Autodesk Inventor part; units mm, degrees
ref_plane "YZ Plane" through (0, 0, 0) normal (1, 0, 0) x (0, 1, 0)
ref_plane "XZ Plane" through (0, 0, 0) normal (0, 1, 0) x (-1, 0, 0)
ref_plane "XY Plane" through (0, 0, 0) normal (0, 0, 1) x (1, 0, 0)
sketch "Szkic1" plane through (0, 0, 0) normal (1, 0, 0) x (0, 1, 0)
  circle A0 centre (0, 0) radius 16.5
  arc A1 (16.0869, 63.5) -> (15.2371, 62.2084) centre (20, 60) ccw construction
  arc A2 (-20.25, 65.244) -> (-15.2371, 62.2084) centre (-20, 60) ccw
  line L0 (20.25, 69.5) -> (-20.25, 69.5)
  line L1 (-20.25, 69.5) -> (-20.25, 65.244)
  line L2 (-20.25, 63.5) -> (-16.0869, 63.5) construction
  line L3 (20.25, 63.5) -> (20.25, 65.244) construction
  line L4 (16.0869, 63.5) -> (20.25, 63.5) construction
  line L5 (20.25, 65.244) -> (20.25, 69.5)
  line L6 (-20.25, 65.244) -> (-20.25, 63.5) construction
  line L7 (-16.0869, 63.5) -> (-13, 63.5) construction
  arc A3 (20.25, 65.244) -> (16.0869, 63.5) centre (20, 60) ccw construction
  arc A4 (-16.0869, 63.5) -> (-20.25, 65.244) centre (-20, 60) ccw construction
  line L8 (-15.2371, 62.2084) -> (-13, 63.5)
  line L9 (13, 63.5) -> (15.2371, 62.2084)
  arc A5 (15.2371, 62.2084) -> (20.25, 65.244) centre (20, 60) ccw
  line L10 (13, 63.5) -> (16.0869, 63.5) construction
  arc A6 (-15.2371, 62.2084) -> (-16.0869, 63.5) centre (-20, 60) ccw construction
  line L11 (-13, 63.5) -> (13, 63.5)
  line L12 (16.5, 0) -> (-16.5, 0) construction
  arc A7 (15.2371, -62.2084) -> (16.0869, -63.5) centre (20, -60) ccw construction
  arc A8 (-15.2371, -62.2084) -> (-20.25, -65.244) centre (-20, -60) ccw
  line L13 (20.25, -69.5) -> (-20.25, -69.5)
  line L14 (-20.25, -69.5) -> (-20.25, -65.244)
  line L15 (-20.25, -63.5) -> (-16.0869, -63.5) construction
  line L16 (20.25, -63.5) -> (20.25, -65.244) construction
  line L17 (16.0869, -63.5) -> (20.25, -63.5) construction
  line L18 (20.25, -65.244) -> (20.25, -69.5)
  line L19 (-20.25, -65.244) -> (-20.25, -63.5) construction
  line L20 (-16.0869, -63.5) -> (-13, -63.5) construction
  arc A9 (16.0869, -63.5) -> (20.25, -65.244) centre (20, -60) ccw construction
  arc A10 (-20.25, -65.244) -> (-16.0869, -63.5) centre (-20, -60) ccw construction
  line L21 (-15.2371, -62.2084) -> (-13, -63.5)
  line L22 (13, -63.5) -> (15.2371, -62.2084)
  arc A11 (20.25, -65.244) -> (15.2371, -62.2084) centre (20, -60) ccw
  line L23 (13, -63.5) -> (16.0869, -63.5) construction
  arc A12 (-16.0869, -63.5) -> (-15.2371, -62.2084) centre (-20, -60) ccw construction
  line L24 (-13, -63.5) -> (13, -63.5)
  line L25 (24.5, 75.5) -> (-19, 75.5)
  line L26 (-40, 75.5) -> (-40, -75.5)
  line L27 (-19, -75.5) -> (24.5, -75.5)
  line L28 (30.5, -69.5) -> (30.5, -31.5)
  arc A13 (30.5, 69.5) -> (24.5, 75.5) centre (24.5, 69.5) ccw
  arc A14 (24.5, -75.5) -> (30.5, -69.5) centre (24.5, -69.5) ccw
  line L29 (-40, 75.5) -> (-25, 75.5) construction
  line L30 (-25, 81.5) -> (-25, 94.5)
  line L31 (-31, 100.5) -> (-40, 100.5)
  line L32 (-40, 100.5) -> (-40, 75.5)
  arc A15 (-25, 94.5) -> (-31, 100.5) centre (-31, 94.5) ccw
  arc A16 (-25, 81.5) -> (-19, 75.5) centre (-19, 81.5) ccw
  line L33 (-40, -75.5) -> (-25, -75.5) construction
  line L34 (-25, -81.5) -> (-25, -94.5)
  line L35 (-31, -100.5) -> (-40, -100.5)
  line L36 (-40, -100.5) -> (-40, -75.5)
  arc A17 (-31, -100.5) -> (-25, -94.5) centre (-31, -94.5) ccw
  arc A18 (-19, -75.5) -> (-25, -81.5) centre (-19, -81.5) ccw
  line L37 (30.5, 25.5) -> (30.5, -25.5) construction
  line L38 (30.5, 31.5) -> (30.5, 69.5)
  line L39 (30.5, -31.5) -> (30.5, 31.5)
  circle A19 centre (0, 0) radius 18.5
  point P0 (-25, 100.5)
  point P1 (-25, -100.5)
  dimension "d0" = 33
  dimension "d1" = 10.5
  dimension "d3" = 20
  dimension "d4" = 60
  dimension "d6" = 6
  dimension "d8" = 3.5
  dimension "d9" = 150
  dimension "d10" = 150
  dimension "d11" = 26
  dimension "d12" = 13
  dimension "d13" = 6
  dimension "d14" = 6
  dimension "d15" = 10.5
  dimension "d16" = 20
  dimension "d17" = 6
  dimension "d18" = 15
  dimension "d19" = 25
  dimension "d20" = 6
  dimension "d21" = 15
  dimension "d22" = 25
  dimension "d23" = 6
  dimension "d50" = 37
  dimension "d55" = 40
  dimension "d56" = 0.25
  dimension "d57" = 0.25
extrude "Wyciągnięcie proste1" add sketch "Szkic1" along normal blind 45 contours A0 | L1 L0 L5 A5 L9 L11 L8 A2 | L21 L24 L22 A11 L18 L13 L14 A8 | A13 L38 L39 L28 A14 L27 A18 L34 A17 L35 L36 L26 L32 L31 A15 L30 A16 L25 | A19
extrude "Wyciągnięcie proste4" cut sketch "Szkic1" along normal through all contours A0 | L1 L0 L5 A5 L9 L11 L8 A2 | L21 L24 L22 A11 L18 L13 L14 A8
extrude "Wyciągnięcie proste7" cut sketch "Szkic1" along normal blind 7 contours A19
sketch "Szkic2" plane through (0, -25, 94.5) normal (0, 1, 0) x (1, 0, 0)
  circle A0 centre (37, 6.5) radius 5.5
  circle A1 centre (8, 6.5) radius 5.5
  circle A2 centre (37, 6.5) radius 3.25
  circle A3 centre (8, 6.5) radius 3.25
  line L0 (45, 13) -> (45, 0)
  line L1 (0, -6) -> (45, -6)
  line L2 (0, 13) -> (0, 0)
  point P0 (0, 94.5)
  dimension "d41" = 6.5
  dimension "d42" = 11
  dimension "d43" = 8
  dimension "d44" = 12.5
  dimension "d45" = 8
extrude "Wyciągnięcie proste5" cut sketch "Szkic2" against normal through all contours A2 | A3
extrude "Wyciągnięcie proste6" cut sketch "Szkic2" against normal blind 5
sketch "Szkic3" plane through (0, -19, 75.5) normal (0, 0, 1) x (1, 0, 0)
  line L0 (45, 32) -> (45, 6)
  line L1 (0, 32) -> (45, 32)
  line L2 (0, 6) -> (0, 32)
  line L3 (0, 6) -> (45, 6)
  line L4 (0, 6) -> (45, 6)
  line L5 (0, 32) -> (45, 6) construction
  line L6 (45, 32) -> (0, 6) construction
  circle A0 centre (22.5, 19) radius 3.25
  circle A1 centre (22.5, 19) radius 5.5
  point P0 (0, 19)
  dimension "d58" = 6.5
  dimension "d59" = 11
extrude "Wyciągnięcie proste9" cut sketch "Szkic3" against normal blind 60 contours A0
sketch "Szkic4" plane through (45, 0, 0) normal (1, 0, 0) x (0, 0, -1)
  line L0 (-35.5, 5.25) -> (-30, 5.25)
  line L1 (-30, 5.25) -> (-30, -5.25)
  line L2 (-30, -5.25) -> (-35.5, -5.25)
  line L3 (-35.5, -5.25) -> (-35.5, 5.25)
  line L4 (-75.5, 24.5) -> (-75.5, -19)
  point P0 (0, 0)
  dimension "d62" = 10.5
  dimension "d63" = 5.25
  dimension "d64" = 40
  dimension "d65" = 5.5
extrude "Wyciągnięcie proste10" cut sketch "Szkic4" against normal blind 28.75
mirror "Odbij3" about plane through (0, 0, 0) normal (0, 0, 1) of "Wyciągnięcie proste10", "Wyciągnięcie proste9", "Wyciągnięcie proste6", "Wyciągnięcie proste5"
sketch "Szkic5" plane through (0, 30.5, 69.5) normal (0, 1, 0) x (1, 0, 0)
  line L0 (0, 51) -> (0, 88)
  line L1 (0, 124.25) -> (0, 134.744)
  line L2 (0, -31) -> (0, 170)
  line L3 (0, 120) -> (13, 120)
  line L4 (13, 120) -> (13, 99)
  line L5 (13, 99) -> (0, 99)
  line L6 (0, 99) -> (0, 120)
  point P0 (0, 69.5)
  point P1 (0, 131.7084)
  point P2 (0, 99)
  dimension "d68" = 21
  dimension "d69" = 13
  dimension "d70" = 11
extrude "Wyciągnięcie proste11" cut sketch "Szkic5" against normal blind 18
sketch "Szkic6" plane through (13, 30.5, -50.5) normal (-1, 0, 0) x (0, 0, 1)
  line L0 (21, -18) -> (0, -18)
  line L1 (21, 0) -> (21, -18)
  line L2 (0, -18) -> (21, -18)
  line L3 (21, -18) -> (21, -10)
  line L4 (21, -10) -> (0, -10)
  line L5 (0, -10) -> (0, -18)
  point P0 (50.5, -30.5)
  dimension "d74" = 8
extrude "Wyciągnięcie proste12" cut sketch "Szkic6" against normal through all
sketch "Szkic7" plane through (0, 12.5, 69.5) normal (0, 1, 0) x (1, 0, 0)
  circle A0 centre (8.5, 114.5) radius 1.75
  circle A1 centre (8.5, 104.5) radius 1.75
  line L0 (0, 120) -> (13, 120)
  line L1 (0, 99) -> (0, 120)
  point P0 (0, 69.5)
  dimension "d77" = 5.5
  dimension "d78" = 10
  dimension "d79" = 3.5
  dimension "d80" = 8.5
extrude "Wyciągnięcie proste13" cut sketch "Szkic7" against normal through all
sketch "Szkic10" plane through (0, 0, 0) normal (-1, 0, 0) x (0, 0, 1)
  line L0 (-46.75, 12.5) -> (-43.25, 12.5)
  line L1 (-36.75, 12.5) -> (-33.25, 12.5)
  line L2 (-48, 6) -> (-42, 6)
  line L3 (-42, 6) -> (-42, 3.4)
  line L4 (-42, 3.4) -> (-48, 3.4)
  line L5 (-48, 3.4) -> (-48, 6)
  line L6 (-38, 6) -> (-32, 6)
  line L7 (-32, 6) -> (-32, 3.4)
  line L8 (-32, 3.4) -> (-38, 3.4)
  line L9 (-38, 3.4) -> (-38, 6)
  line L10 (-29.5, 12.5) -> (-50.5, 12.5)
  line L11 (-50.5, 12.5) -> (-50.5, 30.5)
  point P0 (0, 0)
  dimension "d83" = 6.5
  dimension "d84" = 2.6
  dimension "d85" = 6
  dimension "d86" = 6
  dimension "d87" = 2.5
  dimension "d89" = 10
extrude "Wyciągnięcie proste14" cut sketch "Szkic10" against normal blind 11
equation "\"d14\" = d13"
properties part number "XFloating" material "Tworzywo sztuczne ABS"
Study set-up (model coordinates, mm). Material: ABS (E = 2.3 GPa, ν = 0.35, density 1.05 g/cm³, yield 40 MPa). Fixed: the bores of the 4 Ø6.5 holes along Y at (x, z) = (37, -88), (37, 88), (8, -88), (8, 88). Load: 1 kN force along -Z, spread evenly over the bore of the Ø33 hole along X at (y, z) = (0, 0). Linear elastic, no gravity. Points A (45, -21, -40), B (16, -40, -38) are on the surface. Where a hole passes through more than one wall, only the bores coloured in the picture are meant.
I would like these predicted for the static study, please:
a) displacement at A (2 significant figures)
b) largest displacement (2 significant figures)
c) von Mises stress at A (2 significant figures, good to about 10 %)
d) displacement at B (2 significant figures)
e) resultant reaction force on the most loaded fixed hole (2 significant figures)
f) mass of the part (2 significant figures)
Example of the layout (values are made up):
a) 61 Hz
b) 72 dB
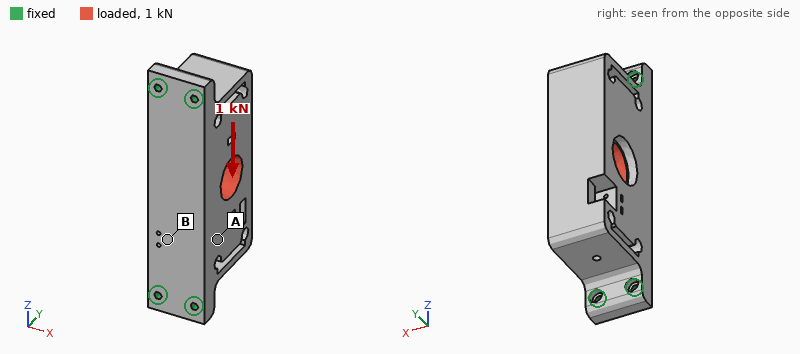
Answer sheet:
a) 26 µm
b) 60 µm
c) 0.62 MPa
d) 21 µm
e) 290 N
f) 430 g
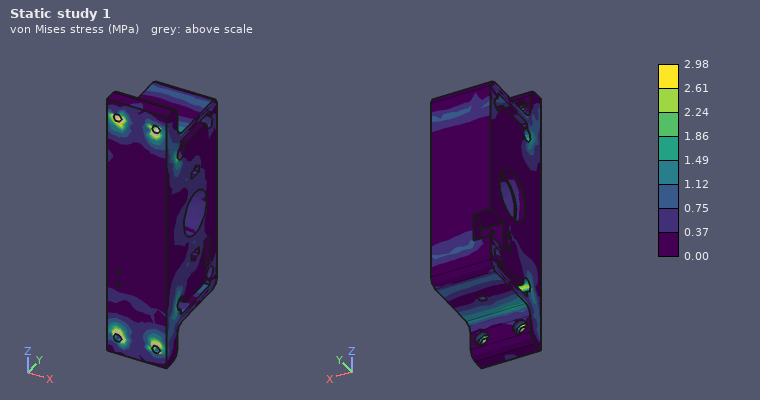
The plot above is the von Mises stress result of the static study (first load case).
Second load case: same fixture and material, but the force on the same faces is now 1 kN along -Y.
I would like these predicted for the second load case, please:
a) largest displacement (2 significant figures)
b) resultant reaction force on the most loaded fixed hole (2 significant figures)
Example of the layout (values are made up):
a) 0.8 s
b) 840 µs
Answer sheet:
a) 0.17 mm
b) 390 N
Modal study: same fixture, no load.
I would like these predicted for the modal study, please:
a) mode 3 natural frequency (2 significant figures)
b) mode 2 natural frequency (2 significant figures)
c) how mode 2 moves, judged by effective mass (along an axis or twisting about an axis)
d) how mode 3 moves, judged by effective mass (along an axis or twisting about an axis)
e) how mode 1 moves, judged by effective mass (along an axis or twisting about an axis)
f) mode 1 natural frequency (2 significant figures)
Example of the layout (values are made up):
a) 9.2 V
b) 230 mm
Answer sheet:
a) 1100 Hz
b) 750 Hz
c) along Y
d) along Z
e) along X
f) 490 Hz
